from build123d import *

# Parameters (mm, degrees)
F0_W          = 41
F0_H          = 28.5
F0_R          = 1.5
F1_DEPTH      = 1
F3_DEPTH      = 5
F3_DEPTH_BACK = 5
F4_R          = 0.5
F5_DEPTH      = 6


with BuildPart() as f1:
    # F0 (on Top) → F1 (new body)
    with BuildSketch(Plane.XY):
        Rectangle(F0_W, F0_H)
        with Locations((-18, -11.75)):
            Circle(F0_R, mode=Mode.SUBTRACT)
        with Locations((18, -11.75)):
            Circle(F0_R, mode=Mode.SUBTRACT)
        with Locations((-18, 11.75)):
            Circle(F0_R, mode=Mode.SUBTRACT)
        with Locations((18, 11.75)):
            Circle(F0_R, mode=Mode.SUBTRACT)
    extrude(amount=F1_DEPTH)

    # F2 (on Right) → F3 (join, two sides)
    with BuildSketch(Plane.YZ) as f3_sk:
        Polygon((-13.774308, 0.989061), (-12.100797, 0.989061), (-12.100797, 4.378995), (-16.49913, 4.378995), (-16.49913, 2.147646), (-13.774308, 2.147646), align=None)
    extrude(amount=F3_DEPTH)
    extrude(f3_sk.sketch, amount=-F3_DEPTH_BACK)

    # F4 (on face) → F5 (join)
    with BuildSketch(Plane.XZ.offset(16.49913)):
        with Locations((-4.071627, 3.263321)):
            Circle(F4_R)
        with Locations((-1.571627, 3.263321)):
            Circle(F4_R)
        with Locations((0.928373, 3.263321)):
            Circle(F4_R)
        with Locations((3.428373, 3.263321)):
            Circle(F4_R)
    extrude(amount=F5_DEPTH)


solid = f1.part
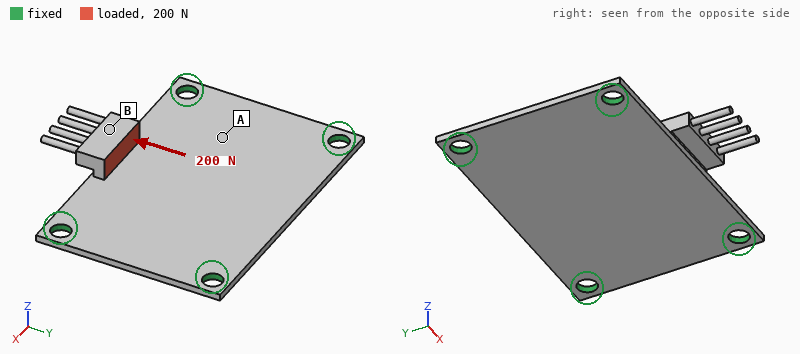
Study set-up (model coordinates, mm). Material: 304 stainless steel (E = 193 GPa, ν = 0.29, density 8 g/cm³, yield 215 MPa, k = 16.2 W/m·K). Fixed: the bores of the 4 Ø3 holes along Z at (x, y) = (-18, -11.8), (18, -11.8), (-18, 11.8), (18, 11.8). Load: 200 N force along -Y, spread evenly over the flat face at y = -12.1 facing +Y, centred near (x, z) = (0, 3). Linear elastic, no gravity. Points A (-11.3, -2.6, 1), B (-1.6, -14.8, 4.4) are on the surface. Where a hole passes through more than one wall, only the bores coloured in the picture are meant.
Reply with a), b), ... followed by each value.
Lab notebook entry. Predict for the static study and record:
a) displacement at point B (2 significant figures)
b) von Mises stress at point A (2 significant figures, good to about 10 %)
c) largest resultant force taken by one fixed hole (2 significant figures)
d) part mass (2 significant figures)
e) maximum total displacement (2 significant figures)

a) 0.056 mm
b) 26 MPa
c) 65 N
d) 10 g
e) 0.12 mm
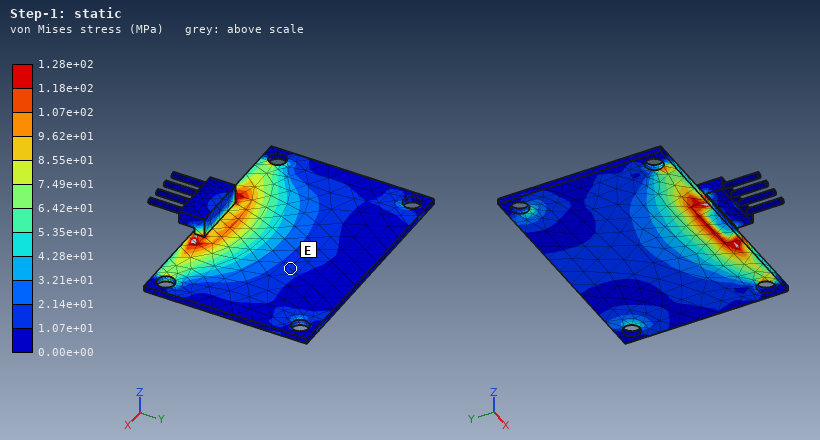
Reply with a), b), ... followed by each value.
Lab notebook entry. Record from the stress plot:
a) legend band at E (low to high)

a) 1.07e+01 to 2.14e+01 MPa
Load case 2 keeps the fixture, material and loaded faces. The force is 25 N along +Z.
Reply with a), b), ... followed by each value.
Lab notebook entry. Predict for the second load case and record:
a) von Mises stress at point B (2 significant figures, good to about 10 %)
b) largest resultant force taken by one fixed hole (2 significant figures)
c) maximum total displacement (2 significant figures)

a) 4.4 MPa
b) 14 N
c) 28 µm
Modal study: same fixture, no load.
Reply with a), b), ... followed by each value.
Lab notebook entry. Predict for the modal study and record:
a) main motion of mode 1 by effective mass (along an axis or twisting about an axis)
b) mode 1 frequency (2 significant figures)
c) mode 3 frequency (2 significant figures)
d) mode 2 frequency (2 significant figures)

a) along Z
b) 3500 Hz
c) 7100 Hz
d) 4200 Hz
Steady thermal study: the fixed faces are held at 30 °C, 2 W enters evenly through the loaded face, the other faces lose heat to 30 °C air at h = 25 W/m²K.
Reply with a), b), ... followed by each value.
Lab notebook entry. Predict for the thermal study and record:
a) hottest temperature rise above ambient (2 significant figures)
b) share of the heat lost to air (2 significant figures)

a) 68 K
b) 51 %
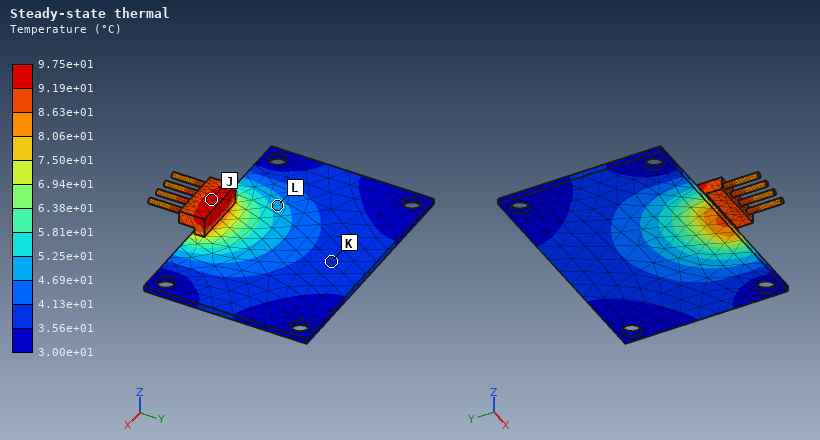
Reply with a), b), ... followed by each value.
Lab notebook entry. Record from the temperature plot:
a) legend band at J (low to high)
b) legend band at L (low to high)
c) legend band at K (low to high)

a) 9.19e+01 to 9.75e+01 °C
b) 4.69e+01 to 5.25e+01 °C
c) 3.56e+01 to 4.13e+01 °C
